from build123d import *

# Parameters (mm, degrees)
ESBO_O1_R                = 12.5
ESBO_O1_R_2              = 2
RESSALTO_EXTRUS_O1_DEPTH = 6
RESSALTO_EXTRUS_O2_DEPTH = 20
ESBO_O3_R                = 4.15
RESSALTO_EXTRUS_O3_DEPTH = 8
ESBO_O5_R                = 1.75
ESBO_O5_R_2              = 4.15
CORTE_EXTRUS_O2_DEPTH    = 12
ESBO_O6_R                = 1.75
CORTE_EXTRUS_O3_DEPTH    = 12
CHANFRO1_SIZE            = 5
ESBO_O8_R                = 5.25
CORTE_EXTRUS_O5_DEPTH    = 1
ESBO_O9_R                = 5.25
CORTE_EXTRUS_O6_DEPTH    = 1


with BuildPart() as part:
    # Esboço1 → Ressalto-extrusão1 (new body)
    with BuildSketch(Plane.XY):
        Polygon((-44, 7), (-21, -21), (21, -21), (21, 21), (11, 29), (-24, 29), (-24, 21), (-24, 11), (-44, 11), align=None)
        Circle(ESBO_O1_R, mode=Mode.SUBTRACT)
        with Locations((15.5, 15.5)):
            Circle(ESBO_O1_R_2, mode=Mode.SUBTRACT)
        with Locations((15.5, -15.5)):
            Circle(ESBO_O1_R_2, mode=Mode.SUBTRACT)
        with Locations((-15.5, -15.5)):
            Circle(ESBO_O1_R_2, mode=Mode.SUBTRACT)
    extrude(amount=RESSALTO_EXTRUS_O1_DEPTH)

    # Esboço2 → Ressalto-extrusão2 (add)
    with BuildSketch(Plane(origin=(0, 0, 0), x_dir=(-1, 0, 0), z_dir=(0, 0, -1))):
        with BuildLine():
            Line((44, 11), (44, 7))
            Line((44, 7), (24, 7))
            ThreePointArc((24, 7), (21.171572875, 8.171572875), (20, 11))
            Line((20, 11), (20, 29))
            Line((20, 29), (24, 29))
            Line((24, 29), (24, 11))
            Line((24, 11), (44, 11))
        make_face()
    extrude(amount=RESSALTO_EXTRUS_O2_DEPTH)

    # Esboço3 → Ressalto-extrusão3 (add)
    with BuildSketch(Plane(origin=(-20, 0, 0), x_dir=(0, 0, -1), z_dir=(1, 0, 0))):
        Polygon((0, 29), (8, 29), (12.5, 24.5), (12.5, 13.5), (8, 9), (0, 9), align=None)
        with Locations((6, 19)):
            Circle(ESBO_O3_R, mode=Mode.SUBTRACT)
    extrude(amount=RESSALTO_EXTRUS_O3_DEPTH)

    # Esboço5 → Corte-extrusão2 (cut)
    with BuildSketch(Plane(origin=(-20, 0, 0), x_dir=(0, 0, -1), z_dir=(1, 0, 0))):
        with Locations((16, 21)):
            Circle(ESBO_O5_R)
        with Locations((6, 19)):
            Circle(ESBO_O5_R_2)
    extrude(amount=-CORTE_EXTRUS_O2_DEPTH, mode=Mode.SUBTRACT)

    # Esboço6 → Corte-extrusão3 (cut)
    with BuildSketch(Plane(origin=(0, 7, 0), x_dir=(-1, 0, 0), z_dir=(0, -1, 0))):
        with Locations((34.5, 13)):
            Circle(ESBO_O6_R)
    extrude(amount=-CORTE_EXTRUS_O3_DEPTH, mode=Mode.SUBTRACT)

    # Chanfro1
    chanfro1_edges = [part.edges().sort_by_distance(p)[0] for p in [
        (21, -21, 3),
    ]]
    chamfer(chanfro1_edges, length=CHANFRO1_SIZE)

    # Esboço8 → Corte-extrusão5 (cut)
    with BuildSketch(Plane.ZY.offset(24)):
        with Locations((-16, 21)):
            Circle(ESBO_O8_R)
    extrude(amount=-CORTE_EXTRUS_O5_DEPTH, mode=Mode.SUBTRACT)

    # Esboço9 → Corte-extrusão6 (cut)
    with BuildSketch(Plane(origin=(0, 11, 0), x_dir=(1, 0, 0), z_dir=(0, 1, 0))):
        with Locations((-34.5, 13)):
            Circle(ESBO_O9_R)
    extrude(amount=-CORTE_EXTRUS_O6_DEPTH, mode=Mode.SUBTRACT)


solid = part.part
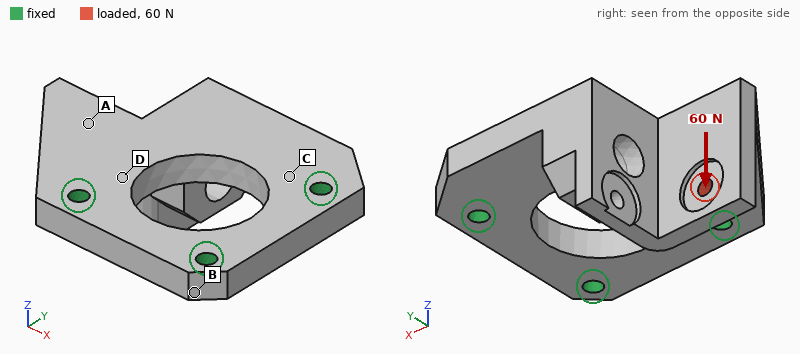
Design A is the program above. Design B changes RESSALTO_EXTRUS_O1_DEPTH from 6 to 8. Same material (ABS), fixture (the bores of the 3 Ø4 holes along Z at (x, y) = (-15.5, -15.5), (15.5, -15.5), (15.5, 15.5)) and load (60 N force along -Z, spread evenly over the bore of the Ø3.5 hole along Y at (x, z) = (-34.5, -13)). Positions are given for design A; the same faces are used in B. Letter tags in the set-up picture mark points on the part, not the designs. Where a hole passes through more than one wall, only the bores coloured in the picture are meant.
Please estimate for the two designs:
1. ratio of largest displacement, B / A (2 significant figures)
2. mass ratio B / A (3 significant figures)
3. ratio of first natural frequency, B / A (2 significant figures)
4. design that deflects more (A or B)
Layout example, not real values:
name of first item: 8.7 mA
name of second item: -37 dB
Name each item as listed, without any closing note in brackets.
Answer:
ratio of largest displacement, B / A: 0.48
mass ratio B / A: 1.25
ratio of first natural frequency, B / A: 1.4
design that deflects more: A
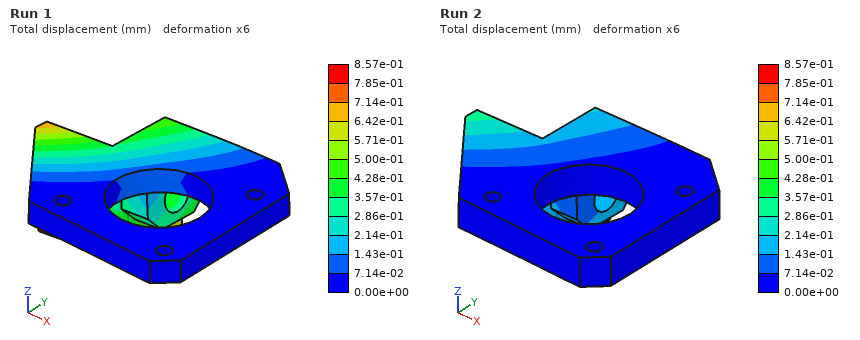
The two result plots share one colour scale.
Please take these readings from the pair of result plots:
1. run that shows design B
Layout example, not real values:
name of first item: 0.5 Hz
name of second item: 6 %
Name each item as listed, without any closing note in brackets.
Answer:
run that shows design B: Run 2
